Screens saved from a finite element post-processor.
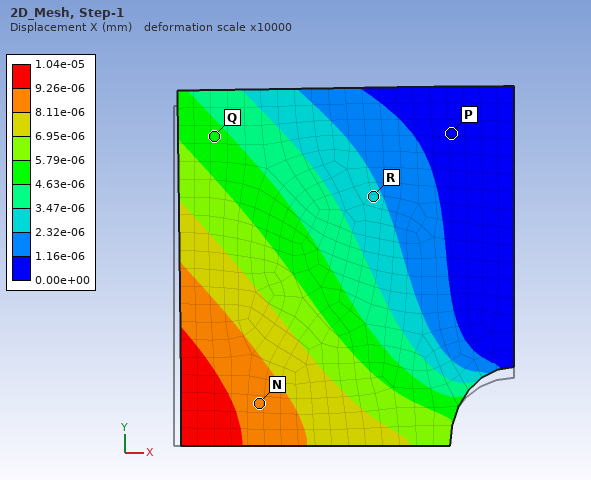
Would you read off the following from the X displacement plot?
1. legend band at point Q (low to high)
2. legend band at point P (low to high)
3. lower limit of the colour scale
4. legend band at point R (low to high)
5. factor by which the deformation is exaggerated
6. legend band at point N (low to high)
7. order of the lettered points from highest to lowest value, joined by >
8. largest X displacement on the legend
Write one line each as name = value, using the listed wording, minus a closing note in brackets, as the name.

legend band at point Q = 4.63e-06 to 5.79e-06 mm
legend band at point P = 0.00e+00 to 1.16e-06 mm
lower limit of the colour scale = 0.00e+00 mm
legend band at point R = 2.32e-06 to 3.47e-06 mm
factor by which the deformation is exaggerated = 10000
legend band at point N = 8.11e-06 to 9.26e-06 mm
order of the lettered points from highest to lowest value, joined by > = N > Q > R > P
largest X displacement on the legend = 1.04e-05 mm
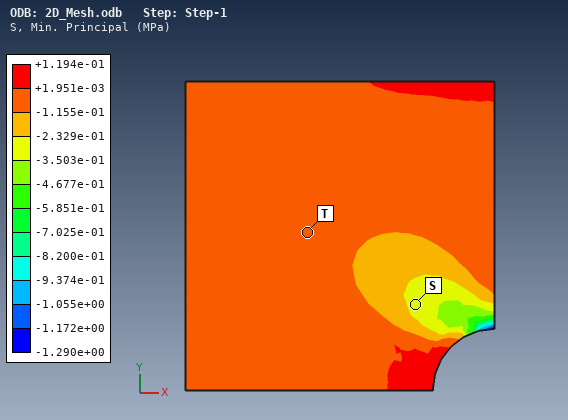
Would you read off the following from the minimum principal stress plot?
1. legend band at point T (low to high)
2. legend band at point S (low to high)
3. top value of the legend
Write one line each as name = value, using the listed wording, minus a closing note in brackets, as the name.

legend band at point T = -1.155e-01 to +1.951e-03 MPa
legend band at point S = -3.503e-01 to -2.329e-01 MPa
top value of the legend = +1.194e-01 MPa
